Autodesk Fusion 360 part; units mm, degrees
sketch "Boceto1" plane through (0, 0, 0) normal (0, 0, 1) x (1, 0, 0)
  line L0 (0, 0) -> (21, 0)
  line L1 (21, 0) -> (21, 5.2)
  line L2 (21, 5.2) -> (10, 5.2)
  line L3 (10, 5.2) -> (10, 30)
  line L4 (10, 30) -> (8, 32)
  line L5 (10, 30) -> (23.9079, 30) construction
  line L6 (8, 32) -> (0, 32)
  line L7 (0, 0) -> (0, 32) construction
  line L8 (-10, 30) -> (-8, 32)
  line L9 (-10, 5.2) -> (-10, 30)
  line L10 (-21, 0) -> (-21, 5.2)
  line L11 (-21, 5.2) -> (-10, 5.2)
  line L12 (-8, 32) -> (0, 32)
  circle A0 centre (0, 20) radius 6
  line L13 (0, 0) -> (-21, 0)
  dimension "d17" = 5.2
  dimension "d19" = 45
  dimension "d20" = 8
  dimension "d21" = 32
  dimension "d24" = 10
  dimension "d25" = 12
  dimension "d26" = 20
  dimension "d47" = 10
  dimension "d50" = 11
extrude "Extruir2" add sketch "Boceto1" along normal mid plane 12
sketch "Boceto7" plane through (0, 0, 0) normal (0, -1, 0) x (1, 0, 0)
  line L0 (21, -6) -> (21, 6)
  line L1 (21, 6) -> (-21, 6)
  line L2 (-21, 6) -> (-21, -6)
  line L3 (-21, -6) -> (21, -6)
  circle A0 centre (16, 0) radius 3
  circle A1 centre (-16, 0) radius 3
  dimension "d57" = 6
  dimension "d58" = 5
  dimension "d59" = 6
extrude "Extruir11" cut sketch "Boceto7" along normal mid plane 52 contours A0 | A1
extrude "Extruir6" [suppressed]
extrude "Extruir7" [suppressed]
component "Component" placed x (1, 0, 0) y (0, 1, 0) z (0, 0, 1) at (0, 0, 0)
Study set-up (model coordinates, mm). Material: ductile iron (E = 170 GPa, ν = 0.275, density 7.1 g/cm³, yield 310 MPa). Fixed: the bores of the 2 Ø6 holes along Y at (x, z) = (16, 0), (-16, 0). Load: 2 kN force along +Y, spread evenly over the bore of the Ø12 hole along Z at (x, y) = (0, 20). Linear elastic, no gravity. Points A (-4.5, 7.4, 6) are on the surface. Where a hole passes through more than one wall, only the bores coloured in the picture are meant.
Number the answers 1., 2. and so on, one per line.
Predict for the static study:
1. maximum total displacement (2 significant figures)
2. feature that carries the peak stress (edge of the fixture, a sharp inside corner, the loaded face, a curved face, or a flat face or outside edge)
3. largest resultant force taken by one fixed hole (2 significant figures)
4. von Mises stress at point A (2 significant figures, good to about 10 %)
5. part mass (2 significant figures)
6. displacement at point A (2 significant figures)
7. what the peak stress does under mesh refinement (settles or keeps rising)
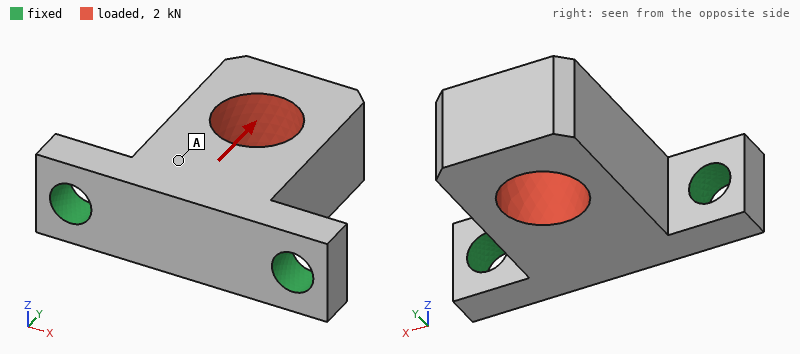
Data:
1. 4.7 µm
2. edge of the fixture
3. 1.1 kN
4. 9.0 MPa
5. 52 g
6. 3.0 µm
7. keeps rising
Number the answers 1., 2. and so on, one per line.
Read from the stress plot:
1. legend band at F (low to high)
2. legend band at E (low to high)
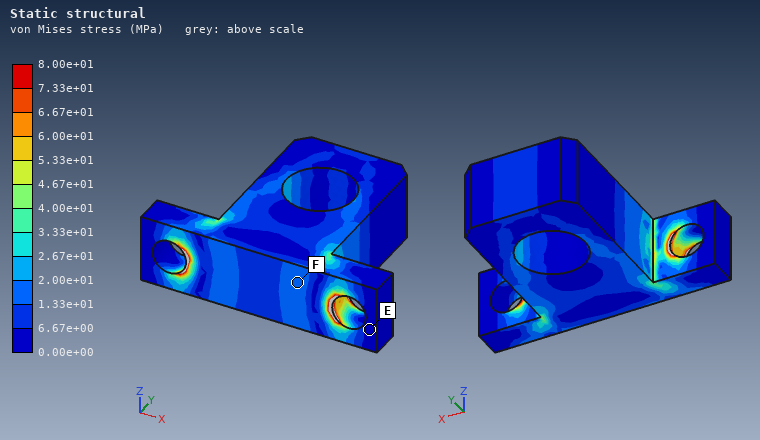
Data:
1. 1.33e+01 to 2.00e+01 MPa
2. 0.00e+00 to 6.67e+00 MPa
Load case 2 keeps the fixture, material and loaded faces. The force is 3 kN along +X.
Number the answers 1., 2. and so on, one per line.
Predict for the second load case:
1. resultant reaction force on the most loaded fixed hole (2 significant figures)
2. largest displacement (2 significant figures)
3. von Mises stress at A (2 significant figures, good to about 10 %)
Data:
1. 2.7 kN
2. 33 µm
3. 29 MPa
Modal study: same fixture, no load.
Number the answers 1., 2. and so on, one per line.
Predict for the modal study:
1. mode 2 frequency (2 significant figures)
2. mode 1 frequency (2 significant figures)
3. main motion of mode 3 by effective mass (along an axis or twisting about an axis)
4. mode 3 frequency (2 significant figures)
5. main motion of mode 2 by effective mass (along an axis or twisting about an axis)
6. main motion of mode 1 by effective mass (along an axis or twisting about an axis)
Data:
1. 9800 Hz
2. 4600 Hz
3. twisting about Y
4. 17 kHz
5. along X
6. along Z
